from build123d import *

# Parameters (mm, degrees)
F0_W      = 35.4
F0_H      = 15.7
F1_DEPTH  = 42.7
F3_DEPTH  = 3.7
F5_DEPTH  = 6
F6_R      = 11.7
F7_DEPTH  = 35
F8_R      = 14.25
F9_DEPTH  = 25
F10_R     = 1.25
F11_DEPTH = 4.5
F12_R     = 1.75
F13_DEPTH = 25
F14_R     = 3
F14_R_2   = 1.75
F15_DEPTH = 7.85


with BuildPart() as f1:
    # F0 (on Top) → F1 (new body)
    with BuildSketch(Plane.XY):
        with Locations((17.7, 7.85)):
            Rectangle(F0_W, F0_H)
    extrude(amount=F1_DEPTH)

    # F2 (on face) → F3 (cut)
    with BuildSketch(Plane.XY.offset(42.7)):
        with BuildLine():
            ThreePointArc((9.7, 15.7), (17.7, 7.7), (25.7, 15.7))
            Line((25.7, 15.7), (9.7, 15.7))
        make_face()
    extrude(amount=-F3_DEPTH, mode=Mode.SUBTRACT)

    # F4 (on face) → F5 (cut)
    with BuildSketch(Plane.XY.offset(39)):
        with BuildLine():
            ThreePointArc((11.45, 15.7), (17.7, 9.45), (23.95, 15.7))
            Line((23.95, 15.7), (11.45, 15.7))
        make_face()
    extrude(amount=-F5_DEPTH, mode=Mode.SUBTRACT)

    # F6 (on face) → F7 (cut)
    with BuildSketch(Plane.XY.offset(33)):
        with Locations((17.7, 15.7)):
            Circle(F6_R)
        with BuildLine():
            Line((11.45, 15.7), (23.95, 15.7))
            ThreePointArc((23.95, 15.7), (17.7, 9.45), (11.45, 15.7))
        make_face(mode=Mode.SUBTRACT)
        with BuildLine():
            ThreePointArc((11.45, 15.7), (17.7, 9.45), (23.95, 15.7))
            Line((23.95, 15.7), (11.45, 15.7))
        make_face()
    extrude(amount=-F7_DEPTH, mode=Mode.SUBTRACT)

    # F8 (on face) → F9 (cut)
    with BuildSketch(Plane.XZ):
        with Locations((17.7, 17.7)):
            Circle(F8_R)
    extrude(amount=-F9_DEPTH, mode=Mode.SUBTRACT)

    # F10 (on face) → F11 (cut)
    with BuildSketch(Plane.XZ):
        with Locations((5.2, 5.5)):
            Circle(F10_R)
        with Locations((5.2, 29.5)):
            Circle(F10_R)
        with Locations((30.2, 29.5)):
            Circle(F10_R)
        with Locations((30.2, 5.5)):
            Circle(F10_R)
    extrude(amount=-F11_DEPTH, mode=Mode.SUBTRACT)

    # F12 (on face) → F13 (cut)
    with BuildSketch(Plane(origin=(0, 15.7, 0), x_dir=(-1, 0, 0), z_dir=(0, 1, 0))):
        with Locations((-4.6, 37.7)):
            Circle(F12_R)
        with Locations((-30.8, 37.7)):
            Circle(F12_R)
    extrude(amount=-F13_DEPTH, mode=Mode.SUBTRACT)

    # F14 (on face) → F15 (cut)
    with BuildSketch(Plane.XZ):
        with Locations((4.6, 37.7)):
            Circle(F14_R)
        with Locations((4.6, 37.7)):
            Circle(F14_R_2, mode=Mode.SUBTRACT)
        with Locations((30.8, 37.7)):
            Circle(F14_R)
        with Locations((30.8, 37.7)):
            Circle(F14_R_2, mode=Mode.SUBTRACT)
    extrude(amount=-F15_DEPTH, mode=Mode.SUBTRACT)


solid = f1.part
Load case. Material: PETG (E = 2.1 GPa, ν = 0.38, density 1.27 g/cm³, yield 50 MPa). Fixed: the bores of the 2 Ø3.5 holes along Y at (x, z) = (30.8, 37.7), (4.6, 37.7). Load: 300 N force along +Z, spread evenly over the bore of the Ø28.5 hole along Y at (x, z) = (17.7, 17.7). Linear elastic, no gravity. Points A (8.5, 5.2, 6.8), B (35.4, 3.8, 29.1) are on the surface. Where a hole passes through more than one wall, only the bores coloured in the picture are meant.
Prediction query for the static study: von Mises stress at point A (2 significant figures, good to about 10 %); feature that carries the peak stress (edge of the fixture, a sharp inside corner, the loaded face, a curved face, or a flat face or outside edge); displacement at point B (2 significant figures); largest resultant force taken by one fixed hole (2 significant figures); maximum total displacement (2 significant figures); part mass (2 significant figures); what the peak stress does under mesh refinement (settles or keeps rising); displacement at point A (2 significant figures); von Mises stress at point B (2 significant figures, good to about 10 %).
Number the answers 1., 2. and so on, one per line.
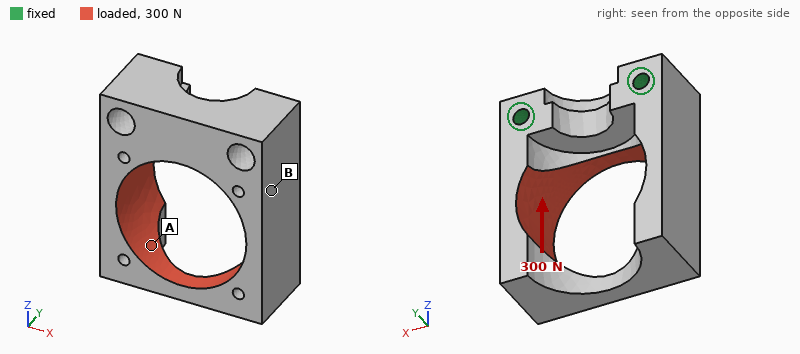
1. 1.1 MPa
2. edge of the fixture
3. 0.048 mm
4. 150 N
5. 0.23 mm
6. 14 g
7. keeps rising
8. 0.15 mm
9. 2.8 MPa
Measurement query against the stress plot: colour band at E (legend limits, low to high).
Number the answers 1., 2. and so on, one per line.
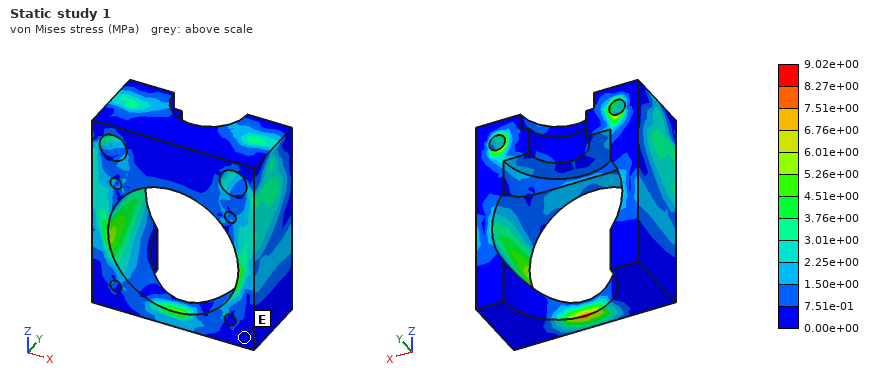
1. 0.00e+00 to 7.51e-01 MPa
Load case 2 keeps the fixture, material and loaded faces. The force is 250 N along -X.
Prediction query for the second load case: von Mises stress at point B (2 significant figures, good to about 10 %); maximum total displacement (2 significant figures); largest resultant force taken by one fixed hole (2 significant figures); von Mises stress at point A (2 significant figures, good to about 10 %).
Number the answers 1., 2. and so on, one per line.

1. 7.0 MPa
2. 0.58 mm
3. 190 N
4. 6.8 MPa
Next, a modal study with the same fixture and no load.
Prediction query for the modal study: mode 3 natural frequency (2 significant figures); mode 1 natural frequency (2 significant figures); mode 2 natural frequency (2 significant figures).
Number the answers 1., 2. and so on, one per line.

1. 2000 Hz
2. 1200 Hz
3. 1200 Hz
